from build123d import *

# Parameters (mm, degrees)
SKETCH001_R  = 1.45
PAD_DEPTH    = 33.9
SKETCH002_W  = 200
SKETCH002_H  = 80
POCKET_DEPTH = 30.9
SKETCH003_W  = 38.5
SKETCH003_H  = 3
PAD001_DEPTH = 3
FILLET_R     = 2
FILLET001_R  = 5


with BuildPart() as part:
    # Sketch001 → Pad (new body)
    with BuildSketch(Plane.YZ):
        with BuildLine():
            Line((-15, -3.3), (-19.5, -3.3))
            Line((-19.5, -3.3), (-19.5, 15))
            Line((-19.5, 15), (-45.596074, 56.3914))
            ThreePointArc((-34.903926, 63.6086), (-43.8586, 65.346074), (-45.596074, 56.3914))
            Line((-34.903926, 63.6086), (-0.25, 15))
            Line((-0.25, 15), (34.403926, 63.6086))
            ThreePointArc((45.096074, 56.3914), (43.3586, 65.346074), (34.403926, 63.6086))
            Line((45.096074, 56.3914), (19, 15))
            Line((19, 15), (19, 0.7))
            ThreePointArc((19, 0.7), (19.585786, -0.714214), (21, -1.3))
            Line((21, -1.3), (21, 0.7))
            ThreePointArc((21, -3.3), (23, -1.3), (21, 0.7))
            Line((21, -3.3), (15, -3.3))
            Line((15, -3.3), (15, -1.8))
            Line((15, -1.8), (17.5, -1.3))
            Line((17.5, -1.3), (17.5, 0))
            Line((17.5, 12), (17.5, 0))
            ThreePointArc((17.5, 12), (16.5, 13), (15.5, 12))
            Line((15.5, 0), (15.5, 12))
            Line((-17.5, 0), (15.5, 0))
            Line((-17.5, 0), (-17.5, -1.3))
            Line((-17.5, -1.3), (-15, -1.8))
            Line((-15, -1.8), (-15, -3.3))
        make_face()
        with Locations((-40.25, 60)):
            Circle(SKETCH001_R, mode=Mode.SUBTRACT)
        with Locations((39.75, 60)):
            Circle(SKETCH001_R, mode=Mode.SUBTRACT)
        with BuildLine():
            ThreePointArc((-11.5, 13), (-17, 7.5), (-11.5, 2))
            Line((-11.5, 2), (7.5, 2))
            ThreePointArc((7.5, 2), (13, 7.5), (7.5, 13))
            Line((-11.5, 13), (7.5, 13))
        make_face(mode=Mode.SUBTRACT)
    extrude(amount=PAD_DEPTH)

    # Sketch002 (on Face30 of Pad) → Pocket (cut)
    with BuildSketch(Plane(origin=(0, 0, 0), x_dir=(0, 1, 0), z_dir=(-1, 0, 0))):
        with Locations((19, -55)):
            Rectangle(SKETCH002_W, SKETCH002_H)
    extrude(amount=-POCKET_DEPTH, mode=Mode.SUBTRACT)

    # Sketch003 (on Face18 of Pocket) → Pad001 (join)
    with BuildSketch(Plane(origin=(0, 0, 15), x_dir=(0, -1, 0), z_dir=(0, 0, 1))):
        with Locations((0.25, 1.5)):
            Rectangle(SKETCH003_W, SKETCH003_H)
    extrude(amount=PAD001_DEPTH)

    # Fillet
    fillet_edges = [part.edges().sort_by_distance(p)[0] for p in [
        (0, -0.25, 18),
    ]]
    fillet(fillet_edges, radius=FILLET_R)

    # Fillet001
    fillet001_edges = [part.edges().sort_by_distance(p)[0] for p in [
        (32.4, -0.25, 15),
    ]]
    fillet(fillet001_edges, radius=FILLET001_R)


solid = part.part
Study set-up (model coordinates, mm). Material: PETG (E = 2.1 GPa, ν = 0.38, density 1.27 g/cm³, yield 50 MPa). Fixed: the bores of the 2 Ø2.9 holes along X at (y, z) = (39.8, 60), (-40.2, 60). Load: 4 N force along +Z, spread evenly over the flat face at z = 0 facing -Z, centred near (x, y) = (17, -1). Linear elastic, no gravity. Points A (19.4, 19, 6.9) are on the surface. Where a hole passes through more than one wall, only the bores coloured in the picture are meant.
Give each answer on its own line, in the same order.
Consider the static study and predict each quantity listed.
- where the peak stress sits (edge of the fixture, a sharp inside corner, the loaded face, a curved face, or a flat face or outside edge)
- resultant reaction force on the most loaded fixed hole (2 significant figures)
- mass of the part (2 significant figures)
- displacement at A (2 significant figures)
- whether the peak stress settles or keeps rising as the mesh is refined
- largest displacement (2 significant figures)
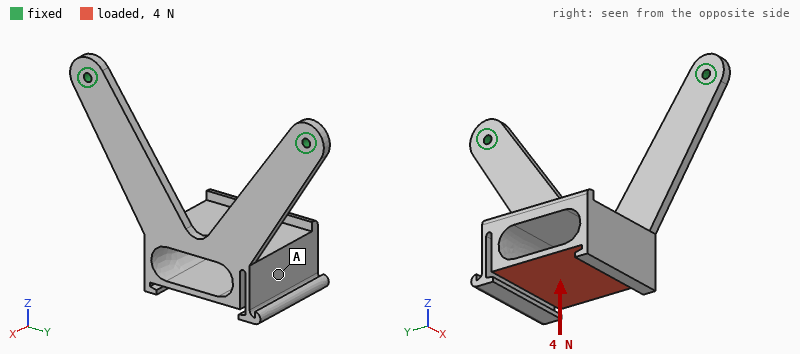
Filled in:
edge of the fixture
2.4 N
19 g
0.77 mm
keeps rising
1.2 mm
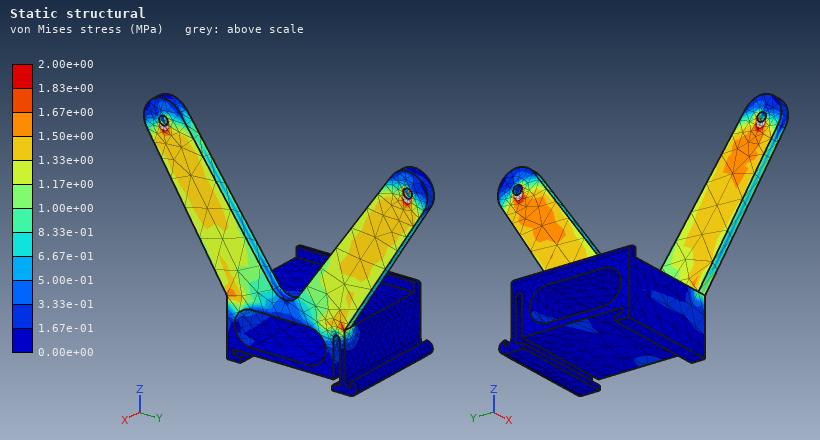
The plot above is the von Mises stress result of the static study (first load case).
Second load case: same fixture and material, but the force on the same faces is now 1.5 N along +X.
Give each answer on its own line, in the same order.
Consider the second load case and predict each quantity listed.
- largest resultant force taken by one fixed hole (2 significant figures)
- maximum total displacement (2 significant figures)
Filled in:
0.78 N
1.2 mm
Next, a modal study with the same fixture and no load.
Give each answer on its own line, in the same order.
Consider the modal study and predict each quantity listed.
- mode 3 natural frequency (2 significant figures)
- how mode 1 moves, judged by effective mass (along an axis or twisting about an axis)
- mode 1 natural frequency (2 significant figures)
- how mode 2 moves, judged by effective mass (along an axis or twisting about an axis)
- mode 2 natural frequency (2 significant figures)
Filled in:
260 Hz
along X
58 Hz
along Y
190 Hz
